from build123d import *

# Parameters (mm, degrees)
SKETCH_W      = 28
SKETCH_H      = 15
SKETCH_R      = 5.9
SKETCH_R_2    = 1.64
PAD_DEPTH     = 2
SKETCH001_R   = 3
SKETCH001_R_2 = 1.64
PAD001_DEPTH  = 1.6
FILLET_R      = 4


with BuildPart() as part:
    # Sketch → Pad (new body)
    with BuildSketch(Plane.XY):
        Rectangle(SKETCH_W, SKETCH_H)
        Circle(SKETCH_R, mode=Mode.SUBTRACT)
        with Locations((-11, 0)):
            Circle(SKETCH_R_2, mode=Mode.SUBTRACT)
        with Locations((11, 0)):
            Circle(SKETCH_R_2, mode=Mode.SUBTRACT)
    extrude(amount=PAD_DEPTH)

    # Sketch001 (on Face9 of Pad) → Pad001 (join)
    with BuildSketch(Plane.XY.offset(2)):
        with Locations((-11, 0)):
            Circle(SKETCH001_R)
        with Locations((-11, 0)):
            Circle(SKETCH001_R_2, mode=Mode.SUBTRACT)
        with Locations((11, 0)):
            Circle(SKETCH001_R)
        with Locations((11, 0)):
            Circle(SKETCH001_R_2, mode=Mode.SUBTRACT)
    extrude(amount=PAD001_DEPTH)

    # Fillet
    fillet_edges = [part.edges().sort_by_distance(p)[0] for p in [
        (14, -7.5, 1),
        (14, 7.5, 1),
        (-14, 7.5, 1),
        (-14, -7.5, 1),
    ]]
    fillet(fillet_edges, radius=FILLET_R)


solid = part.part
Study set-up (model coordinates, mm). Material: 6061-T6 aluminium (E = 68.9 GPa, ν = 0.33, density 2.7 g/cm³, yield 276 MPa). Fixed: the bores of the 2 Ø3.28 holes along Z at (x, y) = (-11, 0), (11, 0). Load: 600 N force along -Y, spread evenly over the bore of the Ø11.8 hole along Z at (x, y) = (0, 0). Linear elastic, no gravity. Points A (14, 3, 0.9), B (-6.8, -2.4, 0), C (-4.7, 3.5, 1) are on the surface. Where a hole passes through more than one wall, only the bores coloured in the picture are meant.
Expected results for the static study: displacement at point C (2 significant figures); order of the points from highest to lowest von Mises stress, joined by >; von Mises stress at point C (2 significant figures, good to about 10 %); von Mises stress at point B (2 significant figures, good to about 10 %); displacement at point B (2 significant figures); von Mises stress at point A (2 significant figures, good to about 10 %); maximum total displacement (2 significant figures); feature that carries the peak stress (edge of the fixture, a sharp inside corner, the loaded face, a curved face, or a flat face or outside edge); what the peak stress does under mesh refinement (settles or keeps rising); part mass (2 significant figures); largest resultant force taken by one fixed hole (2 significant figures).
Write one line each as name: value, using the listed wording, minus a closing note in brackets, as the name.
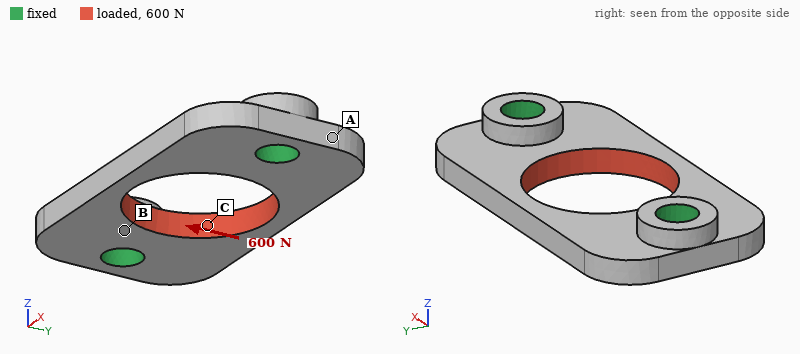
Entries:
displacement at point C: 4.2 µm
order of the points from highest to lowest von Mises stress, joined by >: C > B > A
von Mises stress at point C: 42 MPa
von Mises stress at point B: 28 MPa
displacement at point B: 2.5 µm
von Mises stress at point A: 8.2 MPa
maximum total displacement: 9.0 µm
feature that carries the peak stress: edge of the fixture
what the peak stress does under mesh refinement: keeps rising
part mass: 1.7 g
largest resultant force taken by one fixed hole: 300 N
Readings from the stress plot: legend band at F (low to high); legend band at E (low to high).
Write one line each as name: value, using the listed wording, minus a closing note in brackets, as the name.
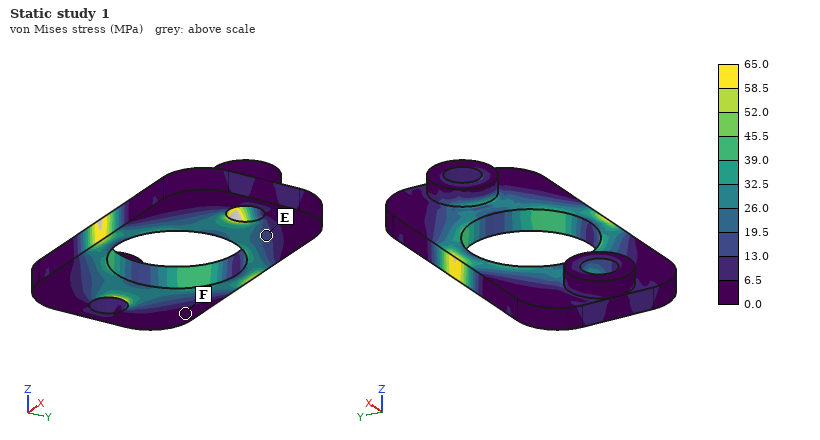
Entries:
legend band at F: 0.0 to 6.5 MPa
legend band at E: 13.0 to 19.5 MPa
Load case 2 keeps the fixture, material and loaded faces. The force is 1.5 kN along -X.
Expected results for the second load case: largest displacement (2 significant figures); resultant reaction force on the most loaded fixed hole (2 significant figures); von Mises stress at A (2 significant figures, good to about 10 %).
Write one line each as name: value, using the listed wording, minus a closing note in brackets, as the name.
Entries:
largest displacement: 8.9 µm
resultant reaction force on the most loaded fixed hole: 750 N
von Mises stress at A: 23 MPa
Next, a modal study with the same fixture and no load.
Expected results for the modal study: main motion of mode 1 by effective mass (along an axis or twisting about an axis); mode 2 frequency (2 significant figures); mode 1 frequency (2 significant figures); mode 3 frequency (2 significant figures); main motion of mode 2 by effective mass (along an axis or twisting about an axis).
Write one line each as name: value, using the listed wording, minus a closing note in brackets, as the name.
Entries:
main motion of mode 1 by effective mass: twisting about X
mode 2 frequency: 24 kHz
mode 1 frequency: 23 kHz
mode 3 frequency: 41 kHz
main motion of mode 2 by effective mass: along Z
